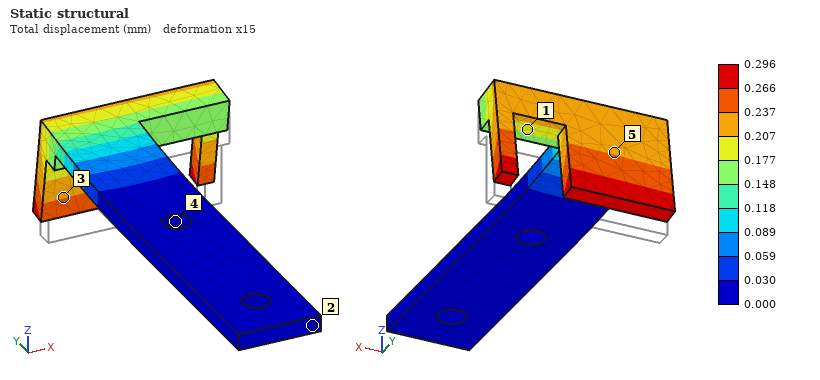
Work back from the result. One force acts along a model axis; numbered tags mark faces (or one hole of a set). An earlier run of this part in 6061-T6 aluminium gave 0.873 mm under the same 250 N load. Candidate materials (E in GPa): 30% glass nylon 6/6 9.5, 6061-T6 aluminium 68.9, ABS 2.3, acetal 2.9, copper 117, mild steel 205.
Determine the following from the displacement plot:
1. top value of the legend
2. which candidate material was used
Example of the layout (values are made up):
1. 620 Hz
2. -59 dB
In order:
1. 0.296 mm
2. mild steel
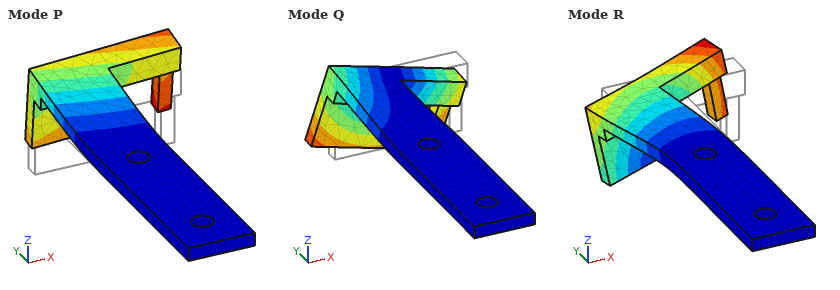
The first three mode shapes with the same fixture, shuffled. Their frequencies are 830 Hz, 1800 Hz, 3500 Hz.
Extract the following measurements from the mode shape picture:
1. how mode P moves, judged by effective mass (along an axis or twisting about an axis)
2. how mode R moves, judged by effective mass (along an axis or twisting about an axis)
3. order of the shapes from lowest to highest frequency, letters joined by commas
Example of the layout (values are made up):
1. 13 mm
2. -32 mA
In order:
1. along Z
2. along X
3. P, Q, R
